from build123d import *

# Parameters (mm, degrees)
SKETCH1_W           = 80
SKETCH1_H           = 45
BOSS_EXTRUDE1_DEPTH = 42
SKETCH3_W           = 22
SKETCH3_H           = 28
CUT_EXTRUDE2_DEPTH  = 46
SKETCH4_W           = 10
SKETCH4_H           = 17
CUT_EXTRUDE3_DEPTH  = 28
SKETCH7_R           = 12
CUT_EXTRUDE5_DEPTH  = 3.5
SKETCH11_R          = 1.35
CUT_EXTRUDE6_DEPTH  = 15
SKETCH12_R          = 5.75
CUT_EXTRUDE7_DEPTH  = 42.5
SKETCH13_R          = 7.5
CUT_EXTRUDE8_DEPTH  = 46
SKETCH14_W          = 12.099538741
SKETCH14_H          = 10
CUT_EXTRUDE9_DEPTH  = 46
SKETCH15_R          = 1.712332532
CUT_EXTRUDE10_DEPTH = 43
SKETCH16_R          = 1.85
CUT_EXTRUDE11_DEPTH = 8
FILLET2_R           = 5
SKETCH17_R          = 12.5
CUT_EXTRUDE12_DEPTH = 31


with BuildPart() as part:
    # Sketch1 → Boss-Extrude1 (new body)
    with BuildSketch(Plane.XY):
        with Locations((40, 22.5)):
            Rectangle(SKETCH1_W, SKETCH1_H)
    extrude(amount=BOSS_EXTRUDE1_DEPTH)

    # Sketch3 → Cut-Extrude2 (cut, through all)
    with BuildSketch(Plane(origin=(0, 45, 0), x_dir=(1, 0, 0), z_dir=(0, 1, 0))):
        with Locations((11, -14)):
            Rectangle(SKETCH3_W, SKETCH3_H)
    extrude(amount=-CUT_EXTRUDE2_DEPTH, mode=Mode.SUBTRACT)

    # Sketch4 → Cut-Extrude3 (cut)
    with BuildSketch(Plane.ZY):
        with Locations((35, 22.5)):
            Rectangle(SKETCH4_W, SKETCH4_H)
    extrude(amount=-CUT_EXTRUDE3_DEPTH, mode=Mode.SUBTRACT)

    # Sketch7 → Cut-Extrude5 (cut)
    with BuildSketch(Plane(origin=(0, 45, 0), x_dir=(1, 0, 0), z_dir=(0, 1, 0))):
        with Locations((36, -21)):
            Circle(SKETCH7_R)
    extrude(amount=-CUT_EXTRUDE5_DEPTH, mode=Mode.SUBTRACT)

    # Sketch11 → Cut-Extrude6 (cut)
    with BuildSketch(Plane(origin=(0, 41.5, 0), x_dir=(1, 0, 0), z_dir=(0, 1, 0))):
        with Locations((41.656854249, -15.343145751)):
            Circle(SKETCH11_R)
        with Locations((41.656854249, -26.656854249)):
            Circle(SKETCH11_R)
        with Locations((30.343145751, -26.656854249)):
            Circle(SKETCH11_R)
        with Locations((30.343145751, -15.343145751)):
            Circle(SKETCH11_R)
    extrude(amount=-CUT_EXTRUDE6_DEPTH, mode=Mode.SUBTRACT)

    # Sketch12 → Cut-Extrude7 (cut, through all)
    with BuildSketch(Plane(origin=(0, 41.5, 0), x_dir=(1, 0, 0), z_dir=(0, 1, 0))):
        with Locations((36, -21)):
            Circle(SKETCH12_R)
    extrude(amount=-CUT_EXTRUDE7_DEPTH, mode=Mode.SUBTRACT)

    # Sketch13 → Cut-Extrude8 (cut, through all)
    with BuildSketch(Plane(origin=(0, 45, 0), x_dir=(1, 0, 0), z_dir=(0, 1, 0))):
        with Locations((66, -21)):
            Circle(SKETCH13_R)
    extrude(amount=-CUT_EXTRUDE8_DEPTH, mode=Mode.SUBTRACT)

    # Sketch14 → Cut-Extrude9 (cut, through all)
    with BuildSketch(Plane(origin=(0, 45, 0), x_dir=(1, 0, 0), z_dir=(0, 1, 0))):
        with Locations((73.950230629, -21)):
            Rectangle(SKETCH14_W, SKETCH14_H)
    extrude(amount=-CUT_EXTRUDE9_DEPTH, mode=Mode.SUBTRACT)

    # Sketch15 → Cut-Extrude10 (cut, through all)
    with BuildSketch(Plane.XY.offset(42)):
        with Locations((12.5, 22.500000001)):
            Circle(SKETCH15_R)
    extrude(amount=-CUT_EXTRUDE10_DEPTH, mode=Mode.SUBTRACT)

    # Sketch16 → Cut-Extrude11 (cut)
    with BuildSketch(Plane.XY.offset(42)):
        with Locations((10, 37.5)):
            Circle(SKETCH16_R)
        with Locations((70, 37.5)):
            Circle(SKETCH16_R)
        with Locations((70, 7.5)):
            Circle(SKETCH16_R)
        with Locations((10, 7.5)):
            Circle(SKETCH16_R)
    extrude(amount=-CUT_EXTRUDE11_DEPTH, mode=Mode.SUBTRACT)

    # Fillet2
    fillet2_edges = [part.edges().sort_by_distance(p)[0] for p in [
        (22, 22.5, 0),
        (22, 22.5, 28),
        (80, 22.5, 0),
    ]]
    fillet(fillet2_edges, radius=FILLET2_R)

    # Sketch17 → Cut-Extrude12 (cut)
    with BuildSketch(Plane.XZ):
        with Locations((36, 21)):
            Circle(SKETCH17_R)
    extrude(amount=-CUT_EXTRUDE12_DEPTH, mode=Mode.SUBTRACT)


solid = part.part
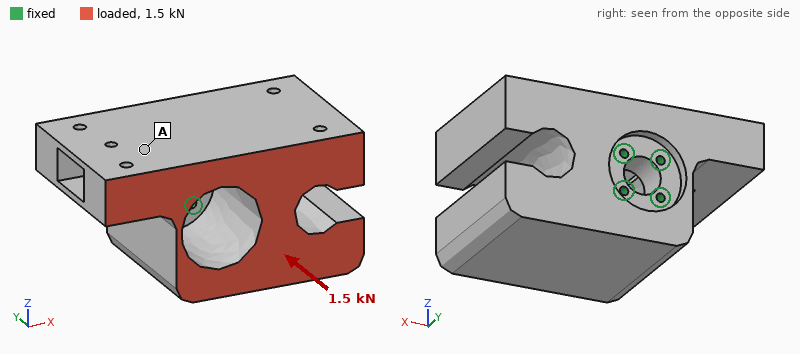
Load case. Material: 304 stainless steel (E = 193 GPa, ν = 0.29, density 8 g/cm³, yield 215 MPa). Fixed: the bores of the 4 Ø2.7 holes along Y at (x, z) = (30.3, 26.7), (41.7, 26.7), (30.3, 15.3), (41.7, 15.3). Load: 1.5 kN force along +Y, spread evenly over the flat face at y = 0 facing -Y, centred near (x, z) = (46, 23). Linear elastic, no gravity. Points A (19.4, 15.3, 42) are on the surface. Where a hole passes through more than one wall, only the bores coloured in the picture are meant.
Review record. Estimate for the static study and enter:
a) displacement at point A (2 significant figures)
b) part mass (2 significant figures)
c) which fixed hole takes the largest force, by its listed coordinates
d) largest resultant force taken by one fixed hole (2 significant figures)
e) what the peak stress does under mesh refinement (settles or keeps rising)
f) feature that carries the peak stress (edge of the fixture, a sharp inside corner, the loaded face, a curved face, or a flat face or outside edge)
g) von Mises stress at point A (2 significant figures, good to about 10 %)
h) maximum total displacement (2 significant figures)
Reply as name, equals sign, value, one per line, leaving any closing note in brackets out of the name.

displacement at point A = 1.1 µm
part mass = 710 g
which fixed hole takes the largest force, by its listed coordinates = (41.7, 26.7)
largest resultant force taken by one fixed hole = 790 N
what the peak stress does under mesh refinement = keeps rising
feature that carries the peak stress = edge of the fixture
von Mises stress at point A = 2.9 MPa
maximum total displacement = 3.7 µm
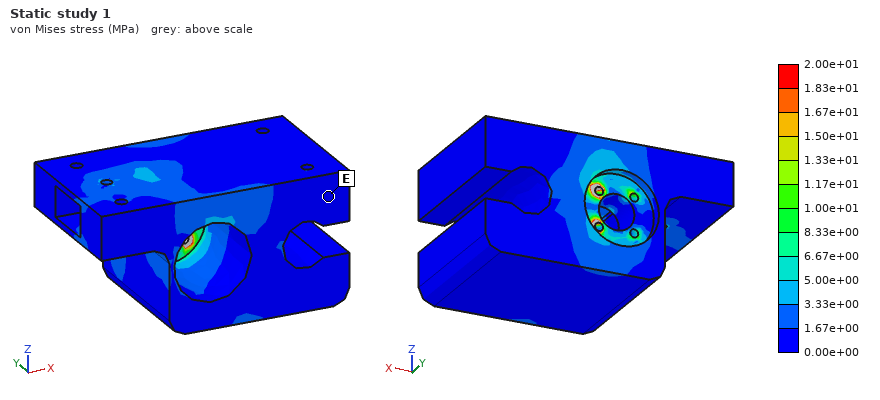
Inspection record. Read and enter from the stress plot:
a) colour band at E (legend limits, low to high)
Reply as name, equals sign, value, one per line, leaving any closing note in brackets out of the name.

colour band at E = 0.00e+00 to 1.67e+00 MPa
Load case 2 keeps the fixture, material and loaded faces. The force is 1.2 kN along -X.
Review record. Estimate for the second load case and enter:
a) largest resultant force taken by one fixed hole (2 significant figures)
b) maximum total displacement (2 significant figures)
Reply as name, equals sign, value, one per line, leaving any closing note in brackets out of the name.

largest resultant force taken by one fixed hole = 1.0 kN
maximum total displacement = 10 µm
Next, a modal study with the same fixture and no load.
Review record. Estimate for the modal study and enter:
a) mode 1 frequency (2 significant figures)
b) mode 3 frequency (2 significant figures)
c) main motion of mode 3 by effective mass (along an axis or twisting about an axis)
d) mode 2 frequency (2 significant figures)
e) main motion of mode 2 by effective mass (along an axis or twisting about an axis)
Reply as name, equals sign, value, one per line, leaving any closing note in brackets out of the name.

mode 1 frequency = 3300 Hz
mode 3 frequency = 5400 Hz
main motion of mode 3 by effective mass = twisting about Y
mode 2 frequency = 4100 Hz
main motion of mode 2 by effective mass = along Z
